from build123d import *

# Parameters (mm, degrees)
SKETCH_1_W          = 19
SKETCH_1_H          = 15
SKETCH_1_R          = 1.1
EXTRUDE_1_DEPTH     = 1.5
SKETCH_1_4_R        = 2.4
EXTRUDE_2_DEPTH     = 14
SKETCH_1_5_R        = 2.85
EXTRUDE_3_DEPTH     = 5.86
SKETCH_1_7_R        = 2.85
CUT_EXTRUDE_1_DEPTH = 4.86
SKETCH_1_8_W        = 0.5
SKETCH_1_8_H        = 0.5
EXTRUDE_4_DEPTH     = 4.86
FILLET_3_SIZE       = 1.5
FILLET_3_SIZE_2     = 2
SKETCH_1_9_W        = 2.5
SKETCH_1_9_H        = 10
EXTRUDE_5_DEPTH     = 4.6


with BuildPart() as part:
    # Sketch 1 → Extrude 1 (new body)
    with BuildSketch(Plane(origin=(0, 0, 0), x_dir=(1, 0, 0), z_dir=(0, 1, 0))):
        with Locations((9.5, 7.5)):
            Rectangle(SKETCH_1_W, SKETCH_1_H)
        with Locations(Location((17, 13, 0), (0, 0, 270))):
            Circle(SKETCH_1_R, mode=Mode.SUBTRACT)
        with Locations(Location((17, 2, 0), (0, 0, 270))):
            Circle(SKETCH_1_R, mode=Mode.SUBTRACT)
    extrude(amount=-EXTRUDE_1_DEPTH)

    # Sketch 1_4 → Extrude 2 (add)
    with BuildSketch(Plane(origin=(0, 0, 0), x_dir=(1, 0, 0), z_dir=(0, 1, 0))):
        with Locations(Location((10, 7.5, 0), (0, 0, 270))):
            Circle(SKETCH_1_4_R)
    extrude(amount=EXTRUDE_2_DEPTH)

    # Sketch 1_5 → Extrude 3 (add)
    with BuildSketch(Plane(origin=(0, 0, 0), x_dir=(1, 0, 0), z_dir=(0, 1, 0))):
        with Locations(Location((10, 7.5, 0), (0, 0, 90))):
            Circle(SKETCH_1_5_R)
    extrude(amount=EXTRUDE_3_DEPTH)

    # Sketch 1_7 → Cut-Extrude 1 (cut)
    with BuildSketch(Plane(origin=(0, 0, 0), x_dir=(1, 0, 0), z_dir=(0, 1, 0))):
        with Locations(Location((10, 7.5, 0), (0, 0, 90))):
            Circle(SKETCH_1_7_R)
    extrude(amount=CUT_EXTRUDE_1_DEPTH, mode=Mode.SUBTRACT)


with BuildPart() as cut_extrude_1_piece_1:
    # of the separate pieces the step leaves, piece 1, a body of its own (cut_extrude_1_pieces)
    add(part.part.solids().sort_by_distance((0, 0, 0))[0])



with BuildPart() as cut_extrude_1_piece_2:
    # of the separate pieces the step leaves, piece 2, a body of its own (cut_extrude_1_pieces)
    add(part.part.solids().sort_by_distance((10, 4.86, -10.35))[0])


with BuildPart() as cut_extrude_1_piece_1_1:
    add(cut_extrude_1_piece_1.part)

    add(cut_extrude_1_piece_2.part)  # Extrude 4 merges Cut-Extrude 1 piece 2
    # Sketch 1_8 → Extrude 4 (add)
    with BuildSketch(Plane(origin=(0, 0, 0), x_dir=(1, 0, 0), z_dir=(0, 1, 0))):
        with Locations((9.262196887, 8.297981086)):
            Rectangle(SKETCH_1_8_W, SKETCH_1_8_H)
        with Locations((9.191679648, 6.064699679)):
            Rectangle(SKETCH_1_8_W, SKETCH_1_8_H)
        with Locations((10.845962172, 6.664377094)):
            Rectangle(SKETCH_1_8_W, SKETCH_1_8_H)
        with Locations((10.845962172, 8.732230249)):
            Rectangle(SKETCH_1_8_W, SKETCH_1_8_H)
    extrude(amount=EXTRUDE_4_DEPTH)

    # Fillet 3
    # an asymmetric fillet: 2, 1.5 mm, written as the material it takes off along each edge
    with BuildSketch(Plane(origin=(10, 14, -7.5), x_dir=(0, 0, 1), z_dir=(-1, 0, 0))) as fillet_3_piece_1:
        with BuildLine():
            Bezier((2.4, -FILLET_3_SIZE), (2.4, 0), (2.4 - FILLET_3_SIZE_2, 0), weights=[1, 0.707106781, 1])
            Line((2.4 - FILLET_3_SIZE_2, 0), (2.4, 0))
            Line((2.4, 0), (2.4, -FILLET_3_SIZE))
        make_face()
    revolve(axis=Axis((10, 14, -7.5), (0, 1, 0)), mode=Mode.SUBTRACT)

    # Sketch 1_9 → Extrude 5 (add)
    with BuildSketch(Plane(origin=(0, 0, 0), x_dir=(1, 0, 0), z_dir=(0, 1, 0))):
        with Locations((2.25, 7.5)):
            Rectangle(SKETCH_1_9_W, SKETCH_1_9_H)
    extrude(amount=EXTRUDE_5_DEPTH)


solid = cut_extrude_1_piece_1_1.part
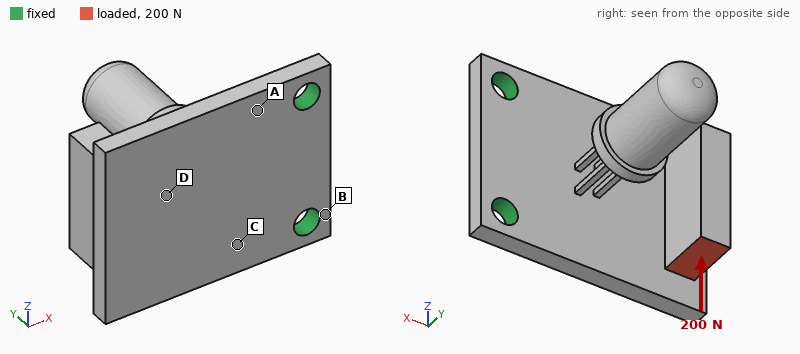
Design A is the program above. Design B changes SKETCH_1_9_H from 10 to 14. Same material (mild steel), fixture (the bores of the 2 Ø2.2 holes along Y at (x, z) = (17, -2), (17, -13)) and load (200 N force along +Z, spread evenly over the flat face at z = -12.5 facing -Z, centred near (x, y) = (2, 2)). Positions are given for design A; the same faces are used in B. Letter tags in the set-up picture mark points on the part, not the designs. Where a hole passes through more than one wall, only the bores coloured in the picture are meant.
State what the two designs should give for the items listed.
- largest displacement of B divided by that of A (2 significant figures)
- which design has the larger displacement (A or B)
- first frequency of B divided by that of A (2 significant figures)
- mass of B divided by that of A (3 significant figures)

1.1
B
1.0
1.07
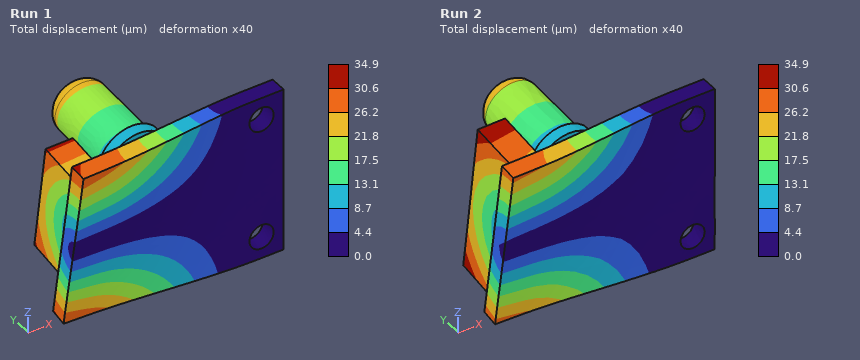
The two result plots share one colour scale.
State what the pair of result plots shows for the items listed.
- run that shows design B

Run 2
